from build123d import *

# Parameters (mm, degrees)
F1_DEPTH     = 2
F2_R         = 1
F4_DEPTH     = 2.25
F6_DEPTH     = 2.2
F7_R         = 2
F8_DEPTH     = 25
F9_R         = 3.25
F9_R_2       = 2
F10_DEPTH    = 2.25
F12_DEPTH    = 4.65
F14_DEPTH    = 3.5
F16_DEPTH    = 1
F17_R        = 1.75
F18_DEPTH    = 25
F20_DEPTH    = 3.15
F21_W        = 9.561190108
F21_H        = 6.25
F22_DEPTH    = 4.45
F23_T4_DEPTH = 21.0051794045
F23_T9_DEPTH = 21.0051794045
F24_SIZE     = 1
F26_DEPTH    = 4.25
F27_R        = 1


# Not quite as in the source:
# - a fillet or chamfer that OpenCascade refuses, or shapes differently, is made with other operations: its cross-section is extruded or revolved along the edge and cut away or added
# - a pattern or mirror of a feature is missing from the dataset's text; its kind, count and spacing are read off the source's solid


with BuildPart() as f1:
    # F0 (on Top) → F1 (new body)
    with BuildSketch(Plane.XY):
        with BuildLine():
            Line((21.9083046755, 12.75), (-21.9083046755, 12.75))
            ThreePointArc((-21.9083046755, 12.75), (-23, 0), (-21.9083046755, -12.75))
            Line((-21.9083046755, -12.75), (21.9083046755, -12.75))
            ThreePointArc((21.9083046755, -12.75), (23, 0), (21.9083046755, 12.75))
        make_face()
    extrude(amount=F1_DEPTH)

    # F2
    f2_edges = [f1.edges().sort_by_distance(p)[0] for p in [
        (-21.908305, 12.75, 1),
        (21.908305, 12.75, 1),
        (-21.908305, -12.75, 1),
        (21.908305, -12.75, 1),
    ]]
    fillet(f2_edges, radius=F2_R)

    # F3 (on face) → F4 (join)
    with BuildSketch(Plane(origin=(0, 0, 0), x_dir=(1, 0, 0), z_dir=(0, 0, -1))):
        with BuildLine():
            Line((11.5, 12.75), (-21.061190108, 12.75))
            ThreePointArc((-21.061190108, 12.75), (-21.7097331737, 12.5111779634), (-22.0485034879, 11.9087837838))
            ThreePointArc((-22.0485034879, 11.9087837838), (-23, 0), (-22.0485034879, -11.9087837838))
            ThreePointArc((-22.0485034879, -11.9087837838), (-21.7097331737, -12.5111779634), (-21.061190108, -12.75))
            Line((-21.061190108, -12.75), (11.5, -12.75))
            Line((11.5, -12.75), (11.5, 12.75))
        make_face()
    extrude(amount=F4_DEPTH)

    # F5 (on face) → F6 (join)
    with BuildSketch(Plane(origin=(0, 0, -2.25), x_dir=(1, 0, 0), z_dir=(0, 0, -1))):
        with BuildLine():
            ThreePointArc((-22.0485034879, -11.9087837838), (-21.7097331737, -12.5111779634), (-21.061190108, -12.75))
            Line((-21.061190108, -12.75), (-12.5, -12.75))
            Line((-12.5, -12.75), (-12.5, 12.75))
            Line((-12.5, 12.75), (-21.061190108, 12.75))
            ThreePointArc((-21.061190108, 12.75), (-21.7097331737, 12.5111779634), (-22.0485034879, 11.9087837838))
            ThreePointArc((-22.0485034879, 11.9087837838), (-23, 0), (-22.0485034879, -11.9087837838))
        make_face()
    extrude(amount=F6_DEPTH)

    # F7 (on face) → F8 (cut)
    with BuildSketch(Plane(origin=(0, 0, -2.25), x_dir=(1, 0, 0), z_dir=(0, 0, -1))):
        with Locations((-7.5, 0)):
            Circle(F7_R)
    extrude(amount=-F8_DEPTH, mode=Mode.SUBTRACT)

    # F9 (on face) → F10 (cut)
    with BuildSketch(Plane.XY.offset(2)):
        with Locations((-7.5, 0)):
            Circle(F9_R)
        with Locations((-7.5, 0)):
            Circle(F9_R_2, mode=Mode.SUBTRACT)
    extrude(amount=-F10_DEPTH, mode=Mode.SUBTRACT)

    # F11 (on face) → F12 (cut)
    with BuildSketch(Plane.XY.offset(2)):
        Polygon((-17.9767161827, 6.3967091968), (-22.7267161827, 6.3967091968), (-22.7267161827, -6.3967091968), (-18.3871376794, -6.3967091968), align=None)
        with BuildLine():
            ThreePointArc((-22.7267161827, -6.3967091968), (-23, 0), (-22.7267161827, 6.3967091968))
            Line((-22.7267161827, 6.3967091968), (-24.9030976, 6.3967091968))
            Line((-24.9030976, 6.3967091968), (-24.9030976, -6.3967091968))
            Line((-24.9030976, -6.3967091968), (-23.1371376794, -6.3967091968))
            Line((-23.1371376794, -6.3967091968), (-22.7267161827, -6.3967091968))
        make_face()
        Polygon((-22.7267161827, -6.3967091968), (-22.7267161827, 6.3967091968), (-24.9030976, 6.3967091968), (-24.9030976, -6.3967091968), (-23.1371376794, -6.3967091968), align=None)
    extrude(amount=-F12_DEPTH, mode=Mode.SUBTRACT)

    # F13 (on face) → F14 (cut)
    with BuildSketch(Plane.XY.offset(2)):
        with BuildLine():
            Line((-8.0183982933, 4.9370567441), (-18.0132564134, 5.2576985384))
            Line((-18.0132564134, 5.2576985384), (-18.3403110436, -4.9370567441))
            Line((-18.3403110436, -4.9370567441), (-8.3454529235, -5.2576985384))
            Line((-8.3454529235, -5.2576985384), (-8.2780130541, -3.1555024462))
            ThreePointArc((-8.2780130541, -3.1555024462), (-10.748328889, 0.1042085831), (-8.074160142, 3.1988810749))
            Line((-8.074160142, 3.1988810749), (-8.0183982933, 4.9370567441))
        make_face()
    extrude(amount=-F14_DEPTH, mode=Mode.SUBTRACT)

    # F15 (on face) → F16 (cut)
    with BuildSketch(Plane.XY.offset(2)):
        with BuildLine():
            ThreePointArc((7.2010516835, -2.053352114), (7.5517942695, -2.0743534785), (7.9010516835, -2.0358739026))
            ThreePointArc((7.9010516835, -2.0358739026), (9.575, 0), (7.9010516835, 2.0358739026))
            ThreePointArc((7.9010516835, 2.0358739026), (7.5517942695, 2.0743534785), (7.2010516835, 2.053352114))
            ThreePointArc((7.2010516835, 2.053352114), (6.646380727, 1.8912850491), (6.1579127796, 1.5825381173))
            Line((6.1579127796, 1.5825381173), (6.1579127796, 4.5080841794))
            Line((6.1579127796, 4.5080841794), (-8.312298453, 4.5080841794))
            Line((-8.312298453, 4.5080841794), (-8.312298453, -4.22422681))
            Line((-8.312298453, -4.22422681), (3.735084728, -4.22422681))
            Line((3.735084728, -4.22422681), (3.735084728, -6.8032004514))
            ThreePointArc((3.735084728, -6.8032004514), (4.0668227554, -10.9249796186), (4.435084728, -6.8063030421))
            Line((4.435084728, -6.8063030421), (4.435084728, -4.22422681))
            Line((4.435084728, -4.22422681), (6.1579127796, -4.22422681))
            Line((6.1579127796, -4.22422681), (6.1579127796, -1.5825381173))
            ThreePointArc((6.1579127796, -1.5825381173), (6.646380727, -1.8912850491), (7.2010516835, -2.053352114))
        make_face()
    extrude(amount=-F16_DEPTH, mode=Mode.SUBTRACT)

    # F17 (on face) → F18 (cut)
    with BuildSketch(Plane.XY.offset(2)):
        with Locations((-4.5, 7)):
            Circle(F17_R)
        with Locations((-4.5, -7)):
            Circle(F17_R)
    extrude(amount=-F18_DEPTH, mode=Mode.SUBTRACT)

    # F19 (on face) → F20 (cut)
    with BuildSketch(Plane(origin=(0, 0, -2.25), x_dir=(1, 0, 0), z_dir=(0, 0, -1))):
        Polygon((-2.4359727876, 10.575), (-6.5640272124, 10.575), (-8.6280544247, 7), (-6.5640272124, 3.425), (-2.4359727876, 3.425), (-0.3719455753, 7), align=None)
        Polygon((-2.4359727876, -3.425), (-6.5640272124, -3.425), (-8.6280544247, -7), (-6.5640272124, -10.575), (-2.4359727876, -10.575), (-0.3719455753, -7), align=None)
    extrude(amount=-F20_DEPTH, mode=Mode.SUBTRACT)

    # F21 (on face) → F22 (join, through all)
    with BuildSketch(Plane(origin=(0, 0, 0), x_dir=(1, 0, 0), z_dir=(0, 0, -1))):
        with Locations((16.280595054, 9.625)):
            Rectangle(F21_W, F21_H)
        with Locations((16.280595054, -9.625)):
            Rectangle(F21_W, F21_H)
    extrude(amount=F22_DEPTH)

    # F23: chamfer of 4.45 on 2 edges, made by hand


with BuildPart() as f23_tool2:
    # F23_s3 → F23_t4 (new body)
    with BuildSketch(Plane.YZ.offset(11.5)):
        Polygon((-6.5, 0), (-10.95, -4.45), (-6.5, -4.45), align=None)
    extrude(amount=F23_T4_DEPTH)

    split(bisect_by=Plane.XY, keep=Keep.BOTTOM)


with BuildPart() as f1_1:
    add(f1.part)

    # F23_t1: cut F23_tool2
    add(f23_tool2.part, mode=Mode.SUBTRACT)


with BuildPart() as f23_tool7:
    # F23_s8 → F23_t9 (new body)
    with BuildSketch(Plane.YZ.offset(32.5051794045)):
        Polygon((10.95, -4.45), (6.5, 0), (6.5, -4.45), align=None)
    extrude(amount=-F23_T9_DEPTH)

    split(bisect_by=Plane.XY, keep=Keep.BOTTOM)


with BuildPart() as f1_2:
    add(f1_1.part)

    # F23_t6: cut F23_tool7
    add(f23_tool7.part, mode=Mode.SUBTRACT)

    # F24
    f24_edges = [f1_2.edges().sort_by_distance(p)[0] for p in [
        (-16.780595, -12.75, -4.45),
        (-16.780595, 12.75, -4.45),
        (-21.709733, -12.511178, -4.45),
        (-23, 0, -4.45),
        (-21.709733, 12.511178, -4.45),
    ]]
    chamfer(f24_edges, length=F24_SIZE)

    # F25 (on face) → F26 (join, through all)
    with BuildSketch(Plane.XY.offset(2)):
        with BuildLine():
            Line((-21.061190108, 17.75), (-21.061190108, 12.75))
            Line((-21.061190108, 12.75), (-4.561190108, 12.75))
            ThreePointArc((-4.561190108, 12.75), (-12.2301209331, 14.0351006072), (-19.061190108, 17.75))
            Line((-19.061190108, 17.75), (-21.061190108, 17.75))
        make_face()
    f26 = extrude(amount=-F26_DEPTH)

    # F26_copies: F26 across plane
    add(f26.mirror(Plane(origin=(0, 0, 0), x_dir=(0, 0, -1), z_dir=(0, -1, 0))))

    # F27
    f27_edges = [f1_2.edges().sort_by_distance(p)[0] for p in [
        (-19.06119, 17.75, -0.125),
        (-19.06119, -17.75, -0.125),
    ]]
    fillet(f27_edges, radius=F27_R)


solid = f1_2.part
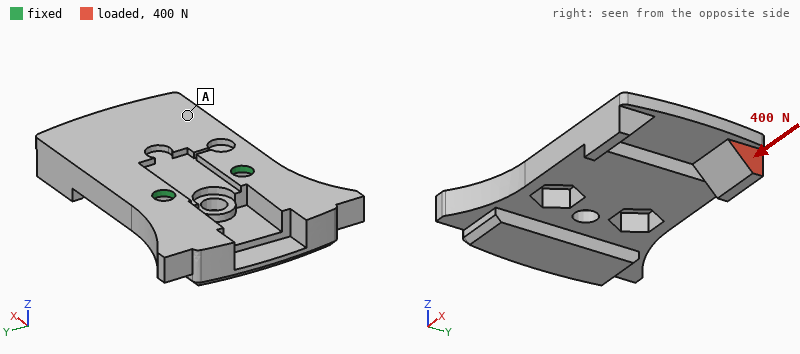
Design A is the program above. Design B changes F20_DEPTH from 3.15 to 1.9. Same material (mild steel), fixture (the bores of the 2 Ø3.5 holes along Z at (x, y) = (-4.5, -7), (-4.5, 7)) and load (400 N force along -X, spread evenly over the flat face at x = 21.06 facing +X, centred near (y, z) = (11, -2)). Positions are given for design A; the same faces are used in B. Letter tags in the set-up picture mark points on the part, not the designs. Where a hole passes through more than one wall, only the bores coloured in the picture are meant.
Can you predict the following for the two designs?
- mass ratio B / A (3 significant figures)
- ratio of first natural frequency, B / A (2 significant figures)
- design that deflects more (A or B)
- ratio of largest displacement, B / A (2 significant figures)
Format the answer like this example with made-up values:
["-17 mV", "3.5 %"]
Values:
["1.02", "1.6", "A", "0.48"]
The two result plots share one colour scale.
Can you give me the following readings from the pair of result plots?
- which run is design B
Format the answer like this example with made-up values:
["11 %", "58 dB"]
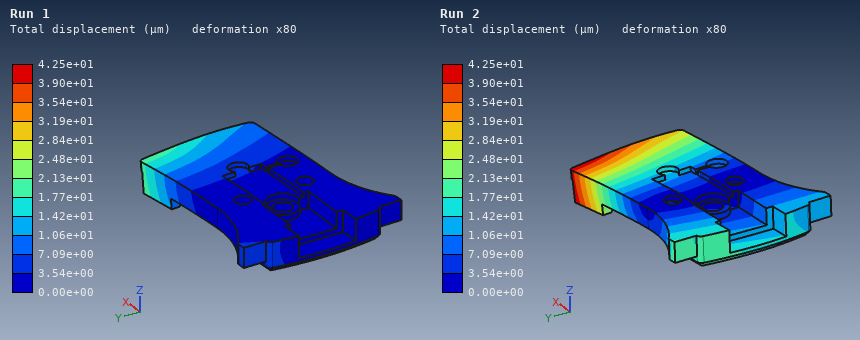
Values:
["Run 1"]
